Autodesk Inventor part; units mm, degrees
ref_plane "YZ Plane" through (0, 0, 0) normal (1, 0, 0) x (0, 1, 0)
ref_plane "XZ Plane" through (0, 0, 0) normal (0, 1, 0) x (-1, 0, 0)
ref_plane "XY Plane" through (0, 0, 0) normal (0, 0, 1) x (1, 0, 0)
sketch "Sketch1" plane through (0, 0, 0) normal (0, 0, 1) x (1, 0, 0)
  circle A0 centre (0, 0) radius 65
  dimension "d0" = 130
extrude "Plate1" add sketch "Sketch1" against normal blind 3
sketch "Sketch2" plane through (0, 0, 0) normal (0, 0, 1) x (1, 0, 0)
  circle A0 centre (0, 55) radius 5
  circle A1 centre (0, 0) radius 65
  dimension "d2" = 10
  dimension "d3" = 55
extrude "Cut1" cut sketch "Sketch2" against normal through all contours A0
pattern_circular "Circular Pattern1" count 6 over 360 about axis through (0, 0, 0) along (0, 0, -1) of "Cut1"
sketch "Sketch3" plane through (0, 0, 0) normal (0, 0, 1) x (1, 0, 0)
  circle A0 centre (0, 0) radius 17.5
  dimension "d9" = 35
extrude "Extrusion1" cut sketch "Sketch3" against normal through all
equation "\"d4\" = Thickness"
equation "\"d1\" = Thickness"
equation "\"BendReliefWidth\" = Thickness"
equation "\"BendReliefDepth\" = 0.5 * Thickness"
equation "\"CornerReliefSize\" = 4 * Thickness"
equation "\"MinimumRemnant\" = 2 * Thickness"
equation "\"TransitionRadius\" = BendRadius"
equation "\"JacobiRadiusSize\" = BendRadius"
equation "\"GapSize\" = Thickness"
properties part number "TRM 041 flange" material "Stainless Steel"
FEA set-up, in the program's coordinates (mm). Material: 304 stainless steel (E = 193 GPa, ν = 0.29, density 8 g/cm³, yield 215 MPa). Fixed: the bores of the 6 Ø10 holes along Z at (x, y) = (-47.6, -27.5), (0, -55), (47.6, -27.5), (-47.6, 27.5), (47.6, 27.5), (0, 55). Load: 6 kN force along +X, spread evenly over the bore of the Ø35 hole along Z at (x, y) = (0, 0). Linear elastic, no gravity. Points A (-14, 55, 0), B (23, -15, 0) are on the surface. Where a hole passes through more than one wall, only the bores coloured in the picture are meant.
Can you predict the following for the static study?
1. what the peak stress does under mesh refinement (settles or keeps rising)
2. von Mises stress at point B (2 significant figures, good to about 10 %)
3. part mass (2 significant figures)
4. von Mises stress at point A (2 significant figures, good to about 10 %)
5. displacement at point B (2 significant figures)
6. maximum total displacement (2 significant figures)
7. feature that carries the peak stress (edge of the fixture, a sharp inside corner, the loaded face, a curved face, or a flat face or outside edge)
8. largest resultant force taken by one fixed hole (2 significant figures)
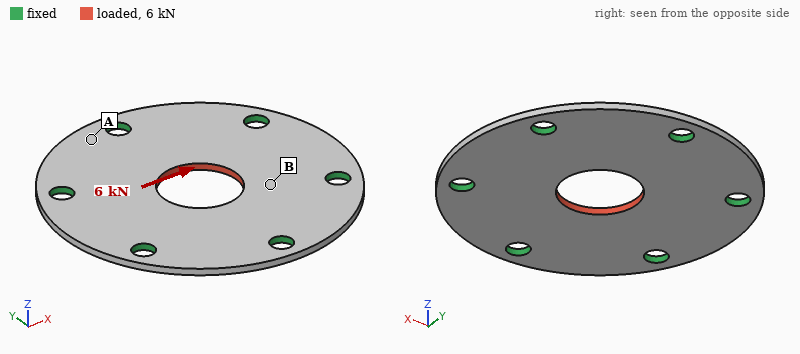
keeps rising
17 MPa
280 g
4.2 MPa
2.4 µm
3.7 µm
edge of the fixture
1.3 kN
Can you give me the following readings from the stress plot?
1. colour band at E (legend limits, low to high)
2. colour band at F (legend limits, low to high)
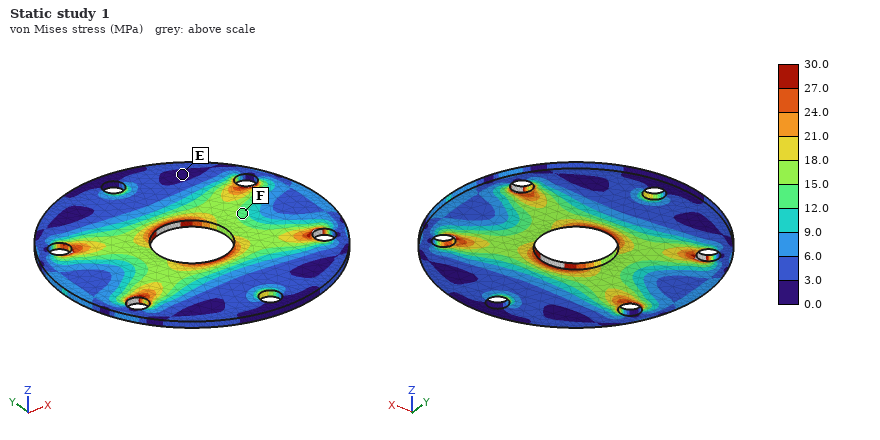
0.0 to 3.0 MPa
12.0 to 15.0 MPa
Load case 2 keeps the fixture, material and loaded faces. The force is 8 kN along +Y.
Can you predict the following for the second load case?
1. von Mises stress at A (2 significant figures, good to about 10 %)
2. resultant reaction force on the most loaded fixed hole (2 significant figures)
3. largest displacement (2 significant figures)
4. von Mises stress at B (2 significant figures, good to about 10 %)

10 MPa
2.0 kN
4.9 µm
17 MPa
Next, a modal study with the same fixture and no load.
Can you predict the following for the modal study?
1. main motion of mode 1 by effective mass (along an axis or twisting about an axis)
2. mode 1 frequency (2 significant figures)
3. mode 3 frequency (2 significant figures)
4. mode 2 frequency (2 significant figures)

along Z
2700 Hz
4300 Hz
4300 Hz
